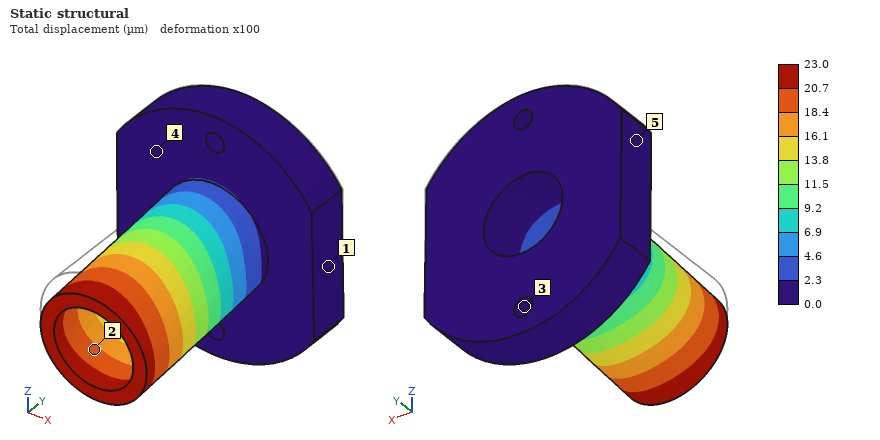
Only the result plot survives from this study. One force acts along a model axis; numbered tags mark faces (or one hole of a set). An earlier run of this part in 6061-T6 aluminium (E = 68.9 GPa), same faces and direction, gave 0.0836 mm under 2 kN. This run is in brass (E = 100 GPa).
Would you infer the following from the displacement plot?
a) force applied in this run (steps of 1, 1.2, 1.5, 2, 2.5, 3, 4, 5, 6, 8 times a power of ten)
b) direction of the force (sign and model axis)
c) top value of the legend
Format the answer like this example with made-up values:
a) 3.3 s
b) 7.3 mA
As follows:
a) 800 N
b) -Z
c) 23.0 µm
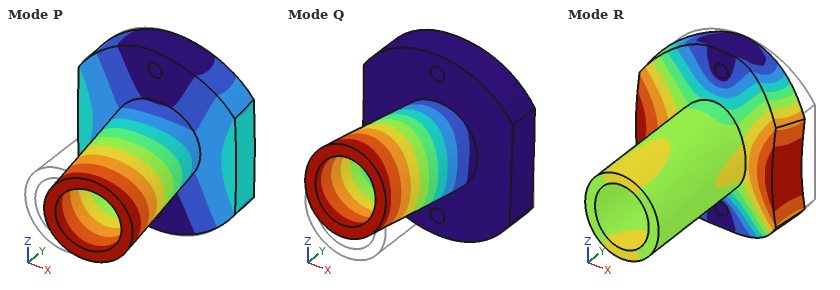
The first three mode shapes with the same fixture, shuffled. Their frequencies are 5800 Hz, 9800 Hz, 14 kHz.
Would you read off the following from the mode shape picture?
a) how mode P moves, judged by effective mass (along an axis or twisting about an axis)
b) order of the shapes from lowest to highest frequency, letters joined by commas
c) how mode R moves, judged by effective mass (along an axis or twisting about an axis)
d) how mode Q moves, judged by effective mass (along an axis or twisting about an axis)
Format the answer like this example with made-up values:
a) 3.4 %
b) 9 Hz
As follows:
a) along X
b) P, Q, R
c) along Y
d) along Z
